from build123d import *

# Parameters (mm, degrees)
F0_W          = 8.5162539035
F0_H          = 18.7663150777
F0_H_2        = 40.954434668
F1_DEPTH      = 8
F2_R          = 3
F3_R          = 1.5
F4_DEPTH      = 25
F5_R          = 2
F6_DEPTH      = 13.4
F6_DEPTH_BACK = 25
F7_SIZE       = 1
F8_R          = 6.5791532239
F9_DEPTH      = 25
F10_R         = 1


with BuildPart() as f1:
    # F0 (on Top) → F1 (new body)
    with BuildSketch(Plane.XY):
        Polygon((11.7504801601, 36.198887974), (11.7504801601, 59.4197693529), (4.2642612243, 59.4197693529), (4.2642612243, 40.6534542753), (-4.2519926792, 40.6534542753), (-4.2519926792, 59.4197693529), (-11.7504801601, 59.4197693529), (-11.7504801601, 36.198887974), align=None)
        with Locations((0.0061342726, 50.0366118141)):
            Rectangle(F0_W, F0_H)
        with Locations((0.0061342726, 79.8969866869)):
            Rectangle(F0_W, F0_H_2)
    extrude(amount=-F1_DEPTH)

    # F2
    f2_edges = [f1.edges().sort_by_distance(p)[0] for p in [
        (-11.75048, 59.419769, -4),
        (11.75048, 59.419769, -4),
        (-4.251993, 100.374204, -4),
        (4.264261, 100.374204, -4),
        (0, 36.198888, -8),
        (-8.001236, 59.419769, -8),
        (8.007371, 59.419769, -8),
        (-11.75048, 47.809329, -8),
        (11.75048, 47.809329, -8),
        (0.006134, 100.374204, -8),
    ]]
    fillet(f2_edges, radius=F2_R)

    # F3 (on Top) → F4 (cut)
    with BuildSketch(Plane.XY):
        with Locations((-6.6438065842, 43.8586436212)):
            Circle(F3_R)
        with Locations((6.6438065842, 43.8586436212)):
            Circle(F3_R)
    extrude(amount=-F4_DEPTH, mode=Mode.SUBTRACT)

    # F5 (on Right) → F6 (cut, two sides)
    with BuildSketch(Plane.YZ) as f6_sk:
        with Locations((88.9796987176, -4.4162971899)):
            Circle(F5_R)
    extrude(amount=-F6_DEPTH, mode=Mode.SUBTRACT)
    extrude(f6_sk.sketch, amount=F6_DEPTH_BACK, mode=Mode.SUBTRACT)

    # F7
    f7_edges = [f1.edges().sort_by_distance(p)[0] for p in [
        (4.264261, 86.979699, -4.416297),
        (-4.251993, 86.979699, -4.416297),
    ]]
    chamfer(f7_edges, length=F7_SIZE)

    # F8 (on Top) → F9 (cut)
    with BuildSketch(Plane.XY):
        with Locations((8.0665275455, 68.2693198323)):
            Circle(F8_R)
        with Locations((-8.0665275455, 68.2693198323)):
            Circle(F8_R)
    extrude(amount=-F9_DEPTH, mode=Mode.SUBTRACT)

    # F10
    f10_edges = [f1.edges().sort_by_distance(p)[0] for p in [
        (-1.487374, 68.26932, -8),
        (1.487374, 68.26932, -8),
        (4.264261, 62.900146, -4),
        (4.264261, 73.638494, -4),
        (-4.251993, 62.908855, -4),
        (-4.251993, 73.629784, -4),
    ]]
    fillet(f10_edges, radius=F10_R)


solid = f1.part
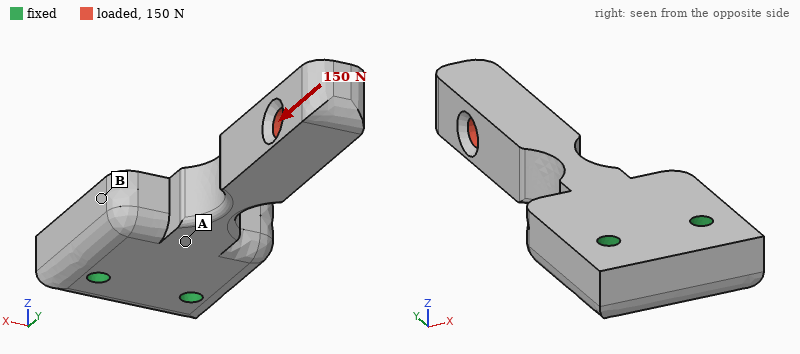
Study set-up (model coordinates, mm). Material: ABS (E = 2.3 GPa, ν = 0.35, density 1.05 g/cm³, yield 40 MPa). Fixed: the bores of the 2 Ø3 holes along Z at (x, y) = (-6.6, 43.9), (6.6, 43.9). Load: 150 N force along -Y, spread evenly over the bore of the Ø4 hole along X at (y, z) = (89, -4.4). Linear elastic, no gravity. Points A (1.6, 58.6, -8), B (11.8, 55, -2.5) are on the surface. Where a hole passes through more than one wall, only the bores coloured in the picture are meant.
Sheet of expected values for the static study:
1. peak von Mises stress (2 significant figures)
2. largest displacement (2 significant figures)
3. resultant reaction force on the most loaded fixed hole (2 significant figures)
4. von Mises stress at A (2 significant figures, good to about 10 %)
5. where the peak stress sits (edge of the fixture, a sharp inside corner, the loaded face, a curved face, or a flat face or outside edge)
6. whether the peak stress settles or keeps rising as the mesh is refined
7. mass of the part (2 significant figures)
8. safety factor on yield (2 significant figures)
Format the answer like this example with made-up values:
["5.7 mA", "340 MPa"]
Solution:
["9.3 MPa", "0.15 mm", "77 N", "2.4 MPa", "a curved face", "settles", "6.7 g", "4.3"]
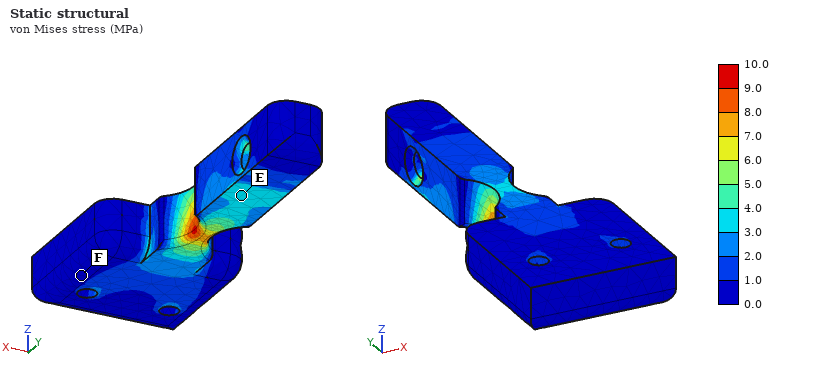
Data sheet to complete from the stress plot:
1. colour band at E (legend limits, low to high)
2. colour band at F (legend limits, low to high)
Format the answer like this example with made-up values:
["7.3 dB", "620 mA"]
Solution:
["3.0 to 4.0 MPa", "0.0 to 1.0 MPa"]
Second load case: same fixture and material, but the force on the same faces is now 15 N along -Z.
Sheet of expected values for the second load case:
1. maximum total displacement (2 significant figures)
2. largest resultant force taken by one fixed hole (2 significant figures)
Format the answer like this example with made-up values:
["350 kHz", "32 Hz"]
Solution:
["0.71 mm", "7.5 N"]
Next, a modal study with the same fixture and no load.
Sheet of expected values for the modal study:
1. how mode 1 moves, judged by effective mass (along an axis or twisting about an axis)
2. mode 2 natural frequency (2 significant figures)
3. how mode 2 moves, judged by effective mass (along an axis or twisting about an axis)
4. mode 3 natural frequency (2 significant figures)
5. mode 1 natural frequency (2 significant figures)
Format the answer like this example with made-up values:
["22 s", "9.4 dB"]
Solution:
["along X", "690 Hz", "along Z", "3200 Hz", "480 Hz"]
